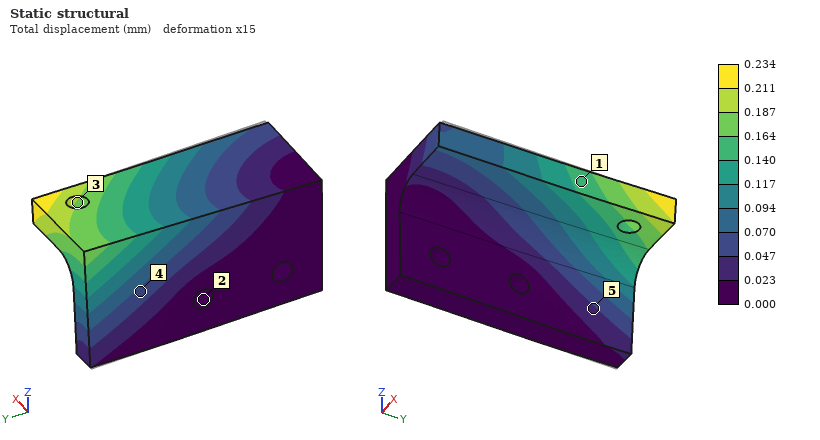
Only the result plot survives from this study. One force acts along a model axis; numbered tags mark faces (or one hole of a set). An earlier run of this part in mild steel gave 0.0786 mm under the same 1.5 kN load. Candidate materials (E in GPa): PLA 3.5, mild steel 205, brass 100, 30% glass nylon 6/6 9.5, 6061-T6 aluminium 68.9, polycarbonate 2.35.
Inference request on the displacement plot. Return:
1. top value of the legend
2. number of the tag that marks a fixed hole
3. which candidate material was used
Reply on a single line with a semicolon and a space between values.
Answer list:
0.234 mm; 2; 6061-T6 aluminium
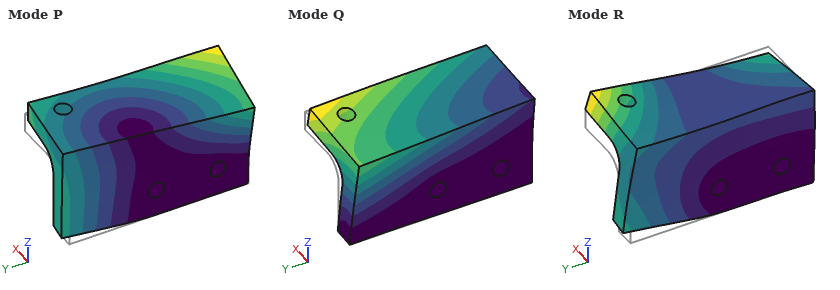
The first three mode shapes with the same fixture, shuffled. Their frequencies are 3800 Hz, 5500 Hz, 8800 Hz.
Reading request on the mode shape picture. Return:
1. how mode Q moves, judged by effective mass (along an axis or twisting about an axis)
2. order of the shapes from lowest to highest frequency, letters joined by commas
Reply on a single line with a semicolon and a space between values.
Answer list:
along X; Q, P, R
